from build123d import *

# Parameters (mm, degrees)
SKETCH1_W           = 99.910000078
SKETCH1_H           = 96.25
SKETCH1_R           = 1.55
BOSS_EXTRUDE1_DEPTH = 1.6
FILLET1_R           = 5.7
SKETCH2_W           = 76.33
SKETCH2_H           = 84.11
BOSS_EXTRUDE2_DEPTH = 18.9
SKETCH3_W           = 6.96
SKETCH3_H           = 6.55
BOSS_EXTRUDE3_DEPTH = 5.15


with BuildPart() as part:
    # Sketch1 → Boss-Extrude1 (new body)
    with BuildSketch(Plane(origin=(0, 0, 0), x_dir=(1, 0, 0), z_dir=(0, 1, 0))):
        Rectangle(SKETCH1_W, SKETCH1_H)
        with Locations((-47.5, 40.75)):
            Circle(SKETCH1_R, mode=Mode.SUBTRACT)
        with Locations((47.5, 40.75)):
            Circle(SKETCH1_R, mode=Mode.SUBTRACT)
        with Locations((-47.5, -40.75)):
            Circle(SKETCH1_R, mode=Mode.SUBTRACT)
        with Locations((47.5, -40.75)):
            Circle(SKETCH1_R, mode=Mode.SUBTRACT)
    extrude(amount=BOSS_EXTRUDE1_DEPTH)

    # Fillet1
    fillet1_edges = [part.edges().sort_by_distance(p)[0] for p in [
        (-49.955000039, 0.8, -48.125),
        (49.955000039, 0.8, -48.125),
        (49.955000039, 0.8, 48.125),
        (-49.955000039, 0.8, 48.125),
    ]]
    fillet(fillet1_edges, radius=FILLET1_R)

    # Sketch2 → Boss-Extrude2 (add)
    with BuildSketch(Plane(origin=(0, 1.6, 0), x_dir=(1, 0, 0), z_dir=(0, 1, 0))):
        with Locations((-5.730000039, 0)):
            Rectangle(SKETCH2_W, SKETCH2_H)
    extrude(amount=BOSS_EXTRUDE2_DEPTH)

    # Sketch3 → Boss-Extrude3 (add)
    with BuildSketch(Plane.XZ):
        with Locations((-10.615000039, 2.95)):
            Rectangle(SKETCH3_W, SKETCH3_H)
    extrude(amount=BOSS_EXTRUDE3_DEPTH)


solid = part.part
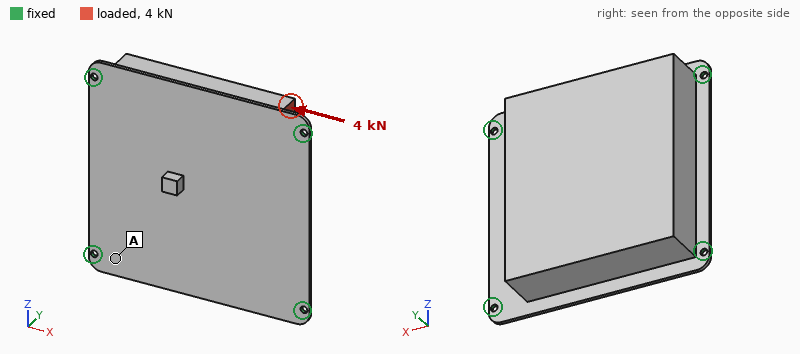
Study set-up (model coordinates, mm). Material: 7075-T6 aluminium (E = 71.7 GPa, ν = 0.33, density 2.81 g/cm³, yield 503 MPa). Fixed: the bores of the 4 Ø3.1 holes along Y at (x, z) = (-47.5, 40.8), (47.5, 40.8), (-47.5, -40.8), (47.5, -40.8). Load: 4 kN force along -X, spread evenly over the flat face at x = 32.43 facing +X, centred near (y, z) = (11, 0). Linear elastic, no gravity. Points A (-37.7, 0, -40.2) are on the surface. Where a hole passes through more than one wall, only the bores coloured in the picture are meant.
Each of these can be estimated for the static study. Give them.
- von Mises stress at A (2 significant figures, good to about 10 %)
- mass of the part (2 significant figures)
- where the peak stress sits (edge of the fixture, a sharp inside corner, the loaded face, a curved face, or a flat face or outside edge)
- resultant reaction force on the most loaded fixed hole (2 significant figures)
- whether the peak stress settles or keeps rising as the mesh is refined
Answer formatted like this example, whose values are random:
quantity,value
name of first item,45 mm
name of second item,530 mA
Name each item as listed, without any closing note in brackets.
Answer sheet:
quantity,value
von Mises stress at A,24 MPa
mass of the part,380 g
where the peak stress sits,edge of the fixture
resultant reaction force on the most loaded fixed hole,1.2 kN
whether the peak stress settles or keeps rising as the mesh is refined,keeps rising
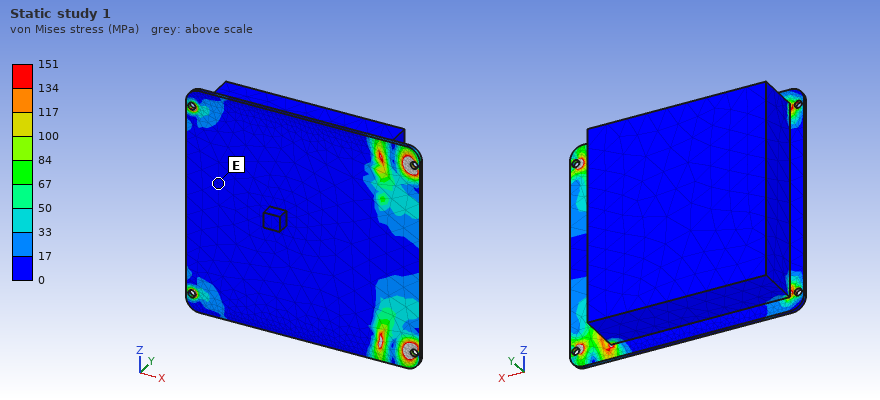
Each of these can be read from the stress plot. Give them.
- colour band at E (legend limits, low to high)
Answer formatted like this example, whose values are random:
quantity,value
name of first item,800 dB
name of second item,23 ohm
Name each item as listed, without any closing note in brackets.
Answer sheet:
quantity,value
colour band at E,0 to 17 MPa
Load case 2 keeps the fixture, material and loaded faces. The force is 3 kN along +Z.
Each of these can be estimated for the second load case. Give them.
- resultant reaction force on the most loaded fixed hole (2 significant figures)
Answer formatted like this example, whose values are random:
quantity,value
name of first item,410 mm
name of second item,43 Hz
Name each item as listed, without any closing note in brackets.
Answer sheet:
quantity,value
resultant reaction force on the most loaded fixed hole,1.1 kN
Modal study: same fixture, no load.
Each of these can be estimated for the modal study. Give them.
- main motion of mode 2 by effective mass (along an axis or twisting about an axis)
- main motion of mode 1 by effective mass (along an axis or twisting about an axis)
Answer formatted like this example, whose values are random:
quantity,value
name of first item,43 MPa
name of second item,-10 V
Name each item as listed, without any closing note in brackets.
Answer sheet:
quantity,value
main motion of mode 2 by effective mass,along Z
main motion of mode 1 by effective mass,along Y
